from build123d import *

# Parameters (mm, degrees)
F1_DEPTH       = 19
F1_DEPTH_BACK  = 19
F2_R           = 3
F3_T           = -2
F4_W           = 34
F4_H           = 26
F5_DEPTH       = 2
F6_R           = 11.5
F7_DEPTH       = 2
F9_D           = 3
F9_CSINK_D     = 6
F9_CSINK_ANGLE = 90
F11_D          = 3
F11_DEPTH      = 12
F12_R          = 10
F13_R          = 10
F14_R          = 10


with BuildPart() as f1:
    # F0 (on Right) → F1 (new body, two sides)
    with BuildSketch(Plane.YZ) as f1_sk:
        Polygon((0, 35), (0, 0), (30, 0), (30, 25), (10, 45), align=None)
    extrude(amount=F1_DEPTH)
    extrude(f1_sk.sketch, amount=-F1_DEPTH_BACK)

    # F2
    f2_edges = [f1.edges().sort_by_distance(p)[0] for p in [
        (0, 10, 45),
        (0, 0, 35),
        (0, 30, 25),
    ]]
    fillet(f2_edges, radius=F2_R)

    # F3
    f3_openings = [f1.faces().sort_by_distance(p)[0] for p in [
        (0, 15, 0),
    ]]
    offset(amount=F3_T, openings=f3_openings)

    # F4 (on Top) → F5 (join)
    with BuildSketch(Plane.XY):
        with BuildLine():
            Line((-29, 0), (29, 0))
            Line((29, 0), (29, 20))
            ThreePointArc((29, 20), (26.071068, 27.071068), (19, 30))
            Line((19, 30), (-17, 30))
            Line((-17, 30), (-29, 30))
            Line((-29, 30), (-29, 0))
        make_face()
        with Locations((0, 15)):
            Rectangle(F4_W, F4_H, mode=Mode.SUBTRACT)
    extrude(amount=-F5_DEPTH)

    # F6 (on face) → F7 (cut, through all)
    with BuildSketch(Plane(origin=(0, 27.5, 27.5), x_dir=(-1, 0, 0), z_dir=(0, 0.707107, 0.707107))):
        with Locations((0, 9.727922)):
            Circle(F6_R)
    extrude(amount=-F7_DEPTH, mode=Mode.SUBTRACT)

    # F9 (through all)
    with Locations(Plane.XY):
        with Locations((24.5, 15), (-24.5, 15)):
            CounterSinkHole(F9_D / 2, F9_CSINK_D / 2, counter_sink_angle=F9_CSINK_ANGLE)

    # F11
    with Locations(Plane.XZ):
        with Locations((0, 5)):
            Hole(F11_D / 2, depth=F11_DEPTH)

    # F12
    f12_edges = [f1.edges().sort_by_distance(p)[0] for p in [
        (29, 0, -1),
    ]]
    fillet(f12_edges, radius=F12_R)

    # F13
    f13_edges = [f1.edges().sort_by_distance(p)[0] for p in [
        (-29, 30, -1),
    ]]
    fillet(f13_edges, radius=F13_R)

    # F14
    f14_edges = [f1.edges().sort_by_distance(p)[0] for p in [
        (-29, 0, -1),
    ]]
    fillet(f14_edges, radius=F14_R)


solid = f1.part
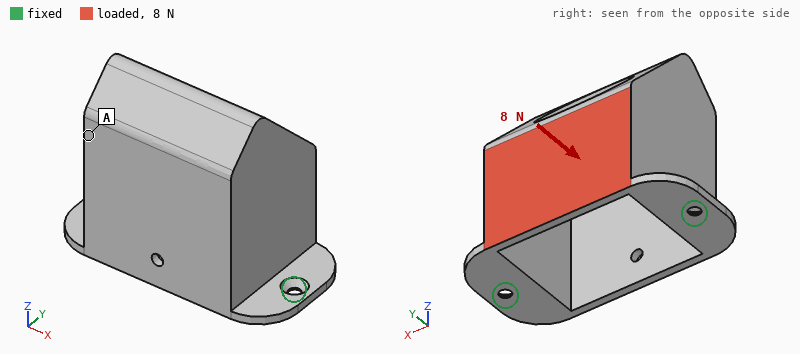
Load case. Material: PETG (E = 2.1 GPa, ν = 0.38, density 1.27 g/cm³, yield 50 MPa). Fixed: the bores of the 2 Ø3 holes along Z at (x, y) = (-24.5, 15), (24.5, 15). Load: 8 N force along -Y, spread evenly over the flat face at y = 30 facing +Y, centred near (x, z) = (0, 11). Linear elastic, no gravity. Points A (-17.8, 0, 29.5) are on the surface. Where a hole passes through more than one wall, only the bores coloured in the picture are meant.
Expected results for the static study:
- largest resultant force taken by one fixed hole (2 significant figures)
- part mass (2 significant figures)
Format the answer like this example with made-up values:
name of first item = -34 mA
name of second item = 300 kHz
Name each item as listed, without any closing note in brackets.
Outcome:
largest resultant force taken by one fixed hole = 4.1 N
part mass = 15 g
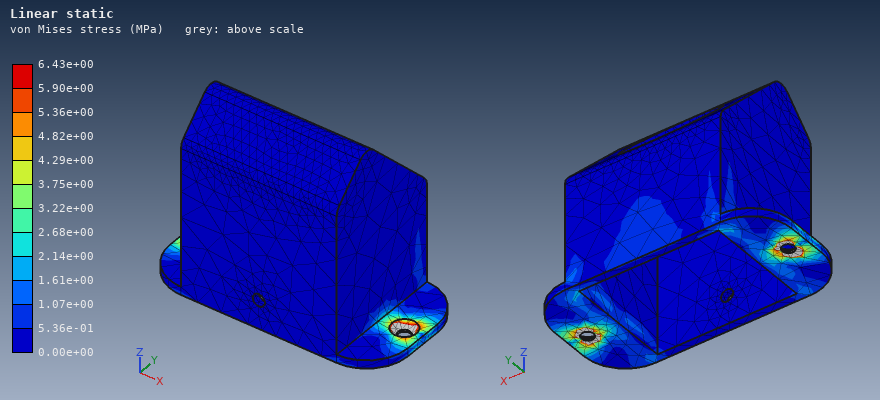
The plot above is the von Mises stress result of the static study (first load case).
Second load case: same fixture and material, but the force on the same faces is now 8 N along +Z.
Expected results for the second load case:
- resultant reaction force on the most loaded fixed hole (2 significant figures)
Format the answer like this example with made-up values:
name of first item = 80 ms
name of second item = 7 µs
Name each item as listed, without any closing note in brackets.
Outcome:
resultant reaction force on the most loaded fixed hole = 4.8 N
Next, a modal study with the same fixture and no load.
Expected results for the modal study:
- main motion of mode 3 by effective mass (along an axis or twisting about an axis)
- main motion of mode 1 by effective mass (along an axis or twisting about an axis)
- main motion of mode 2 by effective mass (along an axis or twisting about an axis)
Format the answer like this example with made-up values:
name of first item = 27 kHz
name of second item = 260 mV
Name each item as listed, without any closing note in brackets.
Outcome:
main motion of mode 3 by effective mass = along Z
main motion of mode 1 by effective mass = along Y
main motion of mode 2 by effective mass = along X
